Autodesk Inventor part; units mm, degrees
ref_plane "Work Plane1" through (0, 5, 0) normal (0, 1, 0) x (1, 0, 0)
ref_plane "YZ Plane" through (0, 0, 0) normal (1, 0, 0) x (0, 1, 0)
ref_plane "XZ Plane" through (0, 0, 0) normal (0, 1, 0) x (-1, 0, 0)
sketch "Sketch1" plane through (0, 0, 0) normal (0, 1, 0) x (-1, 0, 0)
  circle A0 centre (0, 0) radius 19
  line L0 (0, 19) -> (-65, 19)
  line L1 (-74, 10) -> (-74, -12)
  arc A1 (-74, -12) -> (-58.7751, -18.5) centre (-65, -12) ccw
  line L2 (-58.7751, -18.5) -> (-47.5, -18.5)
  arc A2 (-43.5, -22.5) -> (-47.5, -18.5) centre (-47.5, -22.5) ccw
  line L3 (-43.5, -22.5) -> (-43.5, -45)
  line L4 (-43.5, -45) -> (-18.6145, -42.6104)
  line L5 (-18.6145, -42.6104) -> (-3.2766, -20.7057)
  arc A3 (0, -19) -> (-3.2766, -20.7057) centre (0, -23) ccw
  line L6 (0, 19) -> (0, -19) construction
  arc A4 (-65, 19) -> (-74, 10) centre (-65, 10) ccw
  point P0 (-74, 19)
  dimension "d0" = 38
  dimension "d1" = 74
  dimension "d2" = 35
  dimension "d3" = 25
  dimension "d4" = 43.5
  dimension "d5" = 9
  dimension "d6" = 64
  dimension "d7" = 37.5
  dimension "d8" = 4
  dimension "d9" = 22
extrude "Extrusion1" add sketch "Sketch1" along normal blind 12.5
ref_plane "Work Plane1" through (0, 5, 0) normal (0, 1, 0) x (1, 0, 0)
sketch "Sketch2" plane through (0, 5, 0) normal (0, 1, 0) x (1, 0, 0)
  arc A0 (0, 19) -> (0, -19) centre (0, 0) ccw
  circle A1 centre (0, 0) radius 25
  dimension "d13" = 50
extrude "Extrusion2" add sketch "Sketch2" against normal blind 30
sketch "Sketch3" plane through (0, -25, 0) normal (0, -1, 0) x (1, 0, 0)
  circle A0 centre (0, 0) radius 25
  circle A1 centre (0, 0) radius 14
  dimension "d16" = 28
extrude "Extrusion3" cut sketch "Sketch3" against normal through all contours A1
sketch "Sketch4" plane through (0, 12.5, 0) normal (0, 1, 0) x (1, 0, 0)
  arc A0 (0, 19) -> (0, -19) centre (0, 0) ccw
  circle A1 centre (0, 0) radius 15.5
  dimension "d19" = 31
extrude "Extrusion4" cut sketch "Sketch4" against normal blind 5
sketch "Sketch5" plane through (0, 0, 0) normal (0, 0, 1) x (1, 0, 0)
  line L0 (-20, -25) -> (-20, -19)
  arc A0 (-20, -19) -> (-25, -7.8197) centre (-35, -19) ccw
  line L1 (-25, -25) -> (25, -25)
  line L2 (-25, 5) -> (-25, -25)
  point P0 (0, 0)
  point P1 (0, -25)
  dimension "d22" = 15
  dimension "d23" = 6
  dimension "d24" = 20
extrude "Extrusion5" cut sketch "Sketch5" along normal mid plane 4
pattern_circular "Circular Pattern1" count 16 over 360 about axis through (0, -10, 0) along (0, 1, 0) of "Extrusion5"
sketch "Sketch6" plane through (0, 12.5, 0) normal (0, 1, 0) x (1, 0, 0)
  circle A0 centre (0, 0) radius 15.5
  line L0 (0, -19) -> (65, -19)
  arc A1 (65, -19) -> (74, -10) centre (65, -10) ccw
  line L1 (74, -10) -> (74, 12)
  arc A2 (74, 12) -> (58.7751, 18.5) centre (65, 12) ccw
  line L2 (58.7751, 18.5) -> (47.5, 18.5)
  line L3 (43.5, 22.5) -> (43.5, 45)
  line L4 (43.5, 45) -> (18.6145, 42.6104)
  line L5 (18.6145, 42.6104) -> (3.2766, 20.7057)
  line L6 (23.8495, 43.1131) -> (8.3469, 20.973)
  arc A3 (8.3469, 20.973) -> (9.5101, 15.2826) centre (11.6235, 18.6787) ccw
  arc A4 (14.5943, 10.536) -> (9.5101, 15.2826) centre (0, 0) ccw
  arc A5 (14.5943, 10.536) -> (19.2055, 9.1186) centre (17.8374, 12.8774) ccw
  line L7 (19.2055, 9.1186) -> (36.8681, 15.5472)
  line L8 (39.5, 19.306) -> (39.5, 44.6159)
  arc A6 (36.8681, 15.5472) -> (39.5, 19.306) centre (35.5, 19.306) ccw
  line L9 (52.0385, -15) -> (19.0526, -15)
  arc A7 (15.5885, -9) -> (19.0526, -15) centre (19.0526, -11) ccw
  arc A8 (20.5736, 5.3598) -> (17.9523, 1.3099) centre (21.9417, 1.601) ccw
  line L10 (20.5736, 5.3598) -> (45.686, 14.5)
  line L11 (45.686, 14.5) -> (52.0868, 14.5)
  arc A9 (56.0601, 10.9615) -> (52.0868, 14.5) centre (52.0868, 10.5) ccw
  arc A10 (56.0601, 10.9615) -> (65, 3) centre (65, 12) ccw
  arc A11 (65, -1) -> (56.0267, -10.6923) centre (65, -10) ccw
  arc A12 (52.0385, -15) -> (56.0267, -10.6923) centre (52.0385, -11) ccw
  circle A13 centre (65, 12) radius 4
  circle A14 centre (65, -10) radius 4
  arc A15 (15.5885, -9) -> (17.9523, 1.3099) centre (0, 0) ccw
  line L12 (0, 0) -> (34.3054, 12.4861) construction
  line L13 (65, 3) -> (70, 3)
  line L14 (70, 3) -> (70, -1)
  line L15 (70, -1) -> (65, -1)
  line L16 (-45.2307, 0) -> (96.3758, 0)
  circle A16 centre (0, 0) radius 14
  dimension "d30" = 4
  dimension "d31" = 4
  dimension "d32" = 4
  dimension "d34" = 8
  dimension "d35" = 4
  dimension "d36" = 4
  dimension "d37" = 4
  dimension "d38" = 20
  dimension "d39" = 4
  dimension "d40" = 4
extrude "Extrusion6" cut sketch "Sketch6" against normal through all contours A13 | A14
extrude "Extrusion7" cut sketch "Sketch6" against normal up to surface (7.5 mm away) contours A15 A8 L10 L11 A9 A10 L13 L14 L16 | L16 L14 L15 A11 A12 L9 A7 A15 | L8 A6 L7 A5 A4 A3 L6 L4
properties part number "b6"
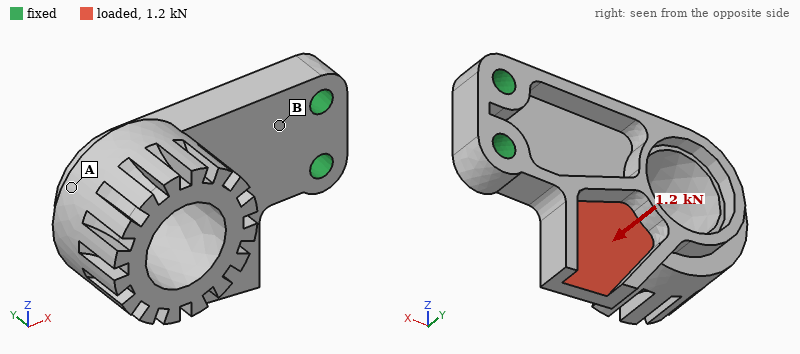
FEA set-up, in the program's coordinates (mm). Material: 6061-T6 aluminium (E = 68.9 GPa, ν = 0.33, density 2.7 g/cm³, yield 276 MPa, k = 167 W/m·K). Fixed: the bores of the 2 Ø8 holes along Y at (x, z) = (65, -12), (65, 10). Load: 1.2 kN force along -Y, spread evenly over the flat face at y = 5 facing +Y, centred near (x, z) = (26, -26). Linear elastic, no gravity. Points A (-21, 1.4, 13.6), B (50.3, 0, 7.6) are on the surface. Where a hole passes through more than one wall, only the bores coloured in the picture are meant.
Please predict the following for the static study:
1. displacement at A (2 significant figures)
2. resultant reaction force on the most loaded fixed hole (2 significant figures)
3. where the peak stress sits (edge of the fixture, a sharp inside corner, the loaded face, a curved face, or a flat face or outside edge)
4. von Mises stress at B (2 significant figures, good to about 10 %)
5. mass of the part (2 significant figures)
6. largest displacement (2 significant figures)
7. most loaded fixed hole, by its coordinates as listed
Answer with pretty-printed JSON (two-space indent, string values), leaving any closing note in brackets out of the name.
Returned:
{
  "displacement at A": "0.26 mm",
  "resultant reaction force on the most loaded fixed hole": "1.6 kN",
  "where the peak stress sits": "a curved face",
  "von Mises stress at B": "36 MPa",
  "mass of the part": "160 g",
  "largest displacement": "0.43 mm",
  "most loaded fixed hole, by its coordinates as listed": "(65, -12)"
}
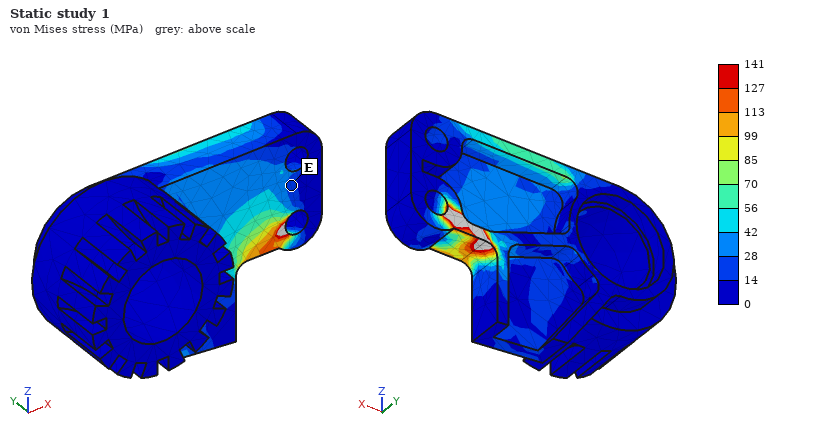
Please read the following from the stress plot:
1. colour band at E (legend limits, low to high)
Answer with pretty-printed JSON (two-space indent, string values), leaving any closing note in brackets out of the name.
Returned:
{
  "colour band at E": "14 to 28 MPa"
}
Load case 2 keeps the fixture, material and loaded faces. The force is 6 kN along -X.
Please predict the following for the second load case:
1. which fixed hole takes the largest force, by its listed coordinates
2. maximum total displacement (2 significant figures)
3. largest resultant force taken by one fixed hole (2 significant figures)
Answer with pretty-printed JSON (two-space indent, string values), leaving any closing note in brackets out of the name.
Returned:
{
  "which fixed hole takes the largest force, by its listed coordinates": "(65, -12)",
  "maximum total displacement": "0.20 mm",
  "largest resultant force taken by one fixed hole": "8.6 kN"
}
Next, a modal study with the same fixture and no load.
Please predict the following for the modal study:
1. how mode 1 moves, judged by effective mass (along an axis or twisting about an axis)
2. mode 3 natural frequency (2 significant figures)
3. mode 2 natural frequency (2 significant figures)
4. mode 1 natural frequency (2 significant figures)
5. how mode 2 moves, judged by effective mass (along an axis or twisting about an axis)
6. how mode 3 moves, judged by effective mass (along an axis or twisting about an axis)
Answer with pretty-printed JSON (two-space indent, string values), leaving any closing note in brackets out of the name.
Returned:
{
  "how mode 1 moves, judged by effective mass": "along Y",
  "mode 3 natural frequency": "2200 Hz",
  "mode 2 natural frequency": "1600 Hz",
  "mode 1 natural frequency": "640 Hz",
  "how mode 2 moves, judged by effective mass": "along Z",
  "how mode 3 moves, judged by effective mass": "along Z"
}
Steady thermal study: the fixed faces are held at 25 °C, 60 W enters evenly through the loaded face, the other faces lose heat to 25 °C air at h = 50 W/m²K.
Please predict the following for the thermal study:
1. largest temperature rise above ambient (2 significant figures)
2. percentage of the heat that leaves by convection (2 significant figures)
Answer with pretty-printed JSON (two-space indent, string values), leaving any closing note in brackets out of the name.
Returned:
{
  "largest temperature rise above ambient": "45 K",
  "percentage of the heat that leaves by convection": "39 %"
}
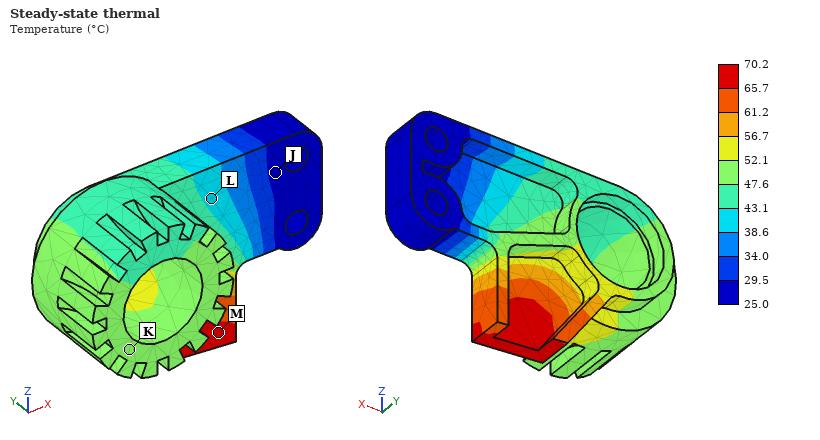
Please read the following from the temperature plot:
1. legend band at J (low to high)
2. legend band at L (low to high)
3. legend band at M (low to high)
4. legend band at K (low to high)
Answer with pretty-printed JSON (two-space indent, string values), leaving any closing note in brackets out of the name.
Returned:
{
  "legend band at J": "25.0 to 29.5 °C",
  "legend band at L": "38.6 to 43.1 °C",
  "legend band at M": "65.7 to 70.2 °C",
  "legend band at K": "47.6 to 52.1 °C"
}
